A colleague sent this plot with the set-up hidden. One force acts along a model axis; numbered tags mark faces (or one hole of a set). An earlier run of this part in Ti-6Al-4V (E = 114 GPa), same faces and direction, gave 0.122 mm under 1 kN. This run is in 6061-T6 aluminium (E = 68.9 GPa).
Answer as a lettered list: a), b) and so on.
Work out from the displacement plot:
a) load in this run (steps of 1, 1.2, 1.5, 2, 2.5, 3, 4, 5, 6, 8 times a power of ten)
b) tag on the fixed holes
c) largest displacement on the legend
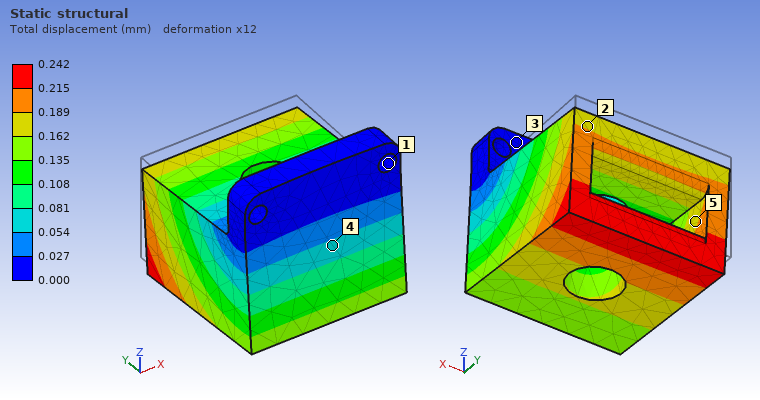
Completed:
a) 1.2 kN
b) 1
c) 0.242 mm
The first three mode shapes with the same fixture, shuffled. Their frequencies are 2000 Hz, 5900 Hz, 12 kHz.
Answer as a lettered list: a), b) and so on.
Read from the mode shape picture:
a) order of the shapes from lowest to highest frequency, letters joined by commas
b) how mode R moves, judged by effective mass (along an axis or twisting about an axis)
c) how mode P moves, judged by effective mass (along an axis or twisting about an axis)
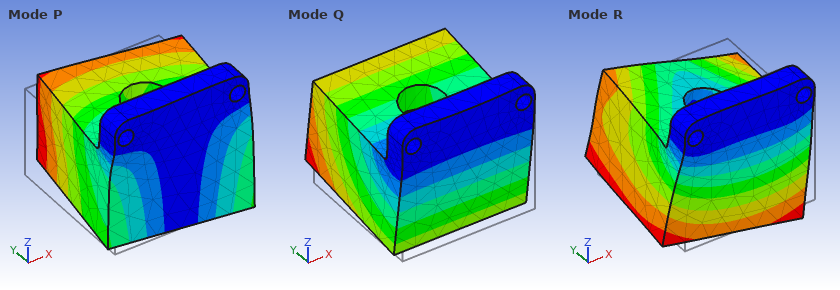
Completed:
a) Q, P, R
b) along X
c) along X
